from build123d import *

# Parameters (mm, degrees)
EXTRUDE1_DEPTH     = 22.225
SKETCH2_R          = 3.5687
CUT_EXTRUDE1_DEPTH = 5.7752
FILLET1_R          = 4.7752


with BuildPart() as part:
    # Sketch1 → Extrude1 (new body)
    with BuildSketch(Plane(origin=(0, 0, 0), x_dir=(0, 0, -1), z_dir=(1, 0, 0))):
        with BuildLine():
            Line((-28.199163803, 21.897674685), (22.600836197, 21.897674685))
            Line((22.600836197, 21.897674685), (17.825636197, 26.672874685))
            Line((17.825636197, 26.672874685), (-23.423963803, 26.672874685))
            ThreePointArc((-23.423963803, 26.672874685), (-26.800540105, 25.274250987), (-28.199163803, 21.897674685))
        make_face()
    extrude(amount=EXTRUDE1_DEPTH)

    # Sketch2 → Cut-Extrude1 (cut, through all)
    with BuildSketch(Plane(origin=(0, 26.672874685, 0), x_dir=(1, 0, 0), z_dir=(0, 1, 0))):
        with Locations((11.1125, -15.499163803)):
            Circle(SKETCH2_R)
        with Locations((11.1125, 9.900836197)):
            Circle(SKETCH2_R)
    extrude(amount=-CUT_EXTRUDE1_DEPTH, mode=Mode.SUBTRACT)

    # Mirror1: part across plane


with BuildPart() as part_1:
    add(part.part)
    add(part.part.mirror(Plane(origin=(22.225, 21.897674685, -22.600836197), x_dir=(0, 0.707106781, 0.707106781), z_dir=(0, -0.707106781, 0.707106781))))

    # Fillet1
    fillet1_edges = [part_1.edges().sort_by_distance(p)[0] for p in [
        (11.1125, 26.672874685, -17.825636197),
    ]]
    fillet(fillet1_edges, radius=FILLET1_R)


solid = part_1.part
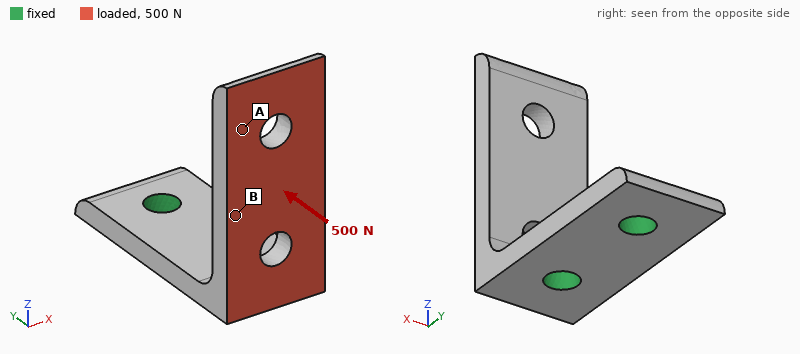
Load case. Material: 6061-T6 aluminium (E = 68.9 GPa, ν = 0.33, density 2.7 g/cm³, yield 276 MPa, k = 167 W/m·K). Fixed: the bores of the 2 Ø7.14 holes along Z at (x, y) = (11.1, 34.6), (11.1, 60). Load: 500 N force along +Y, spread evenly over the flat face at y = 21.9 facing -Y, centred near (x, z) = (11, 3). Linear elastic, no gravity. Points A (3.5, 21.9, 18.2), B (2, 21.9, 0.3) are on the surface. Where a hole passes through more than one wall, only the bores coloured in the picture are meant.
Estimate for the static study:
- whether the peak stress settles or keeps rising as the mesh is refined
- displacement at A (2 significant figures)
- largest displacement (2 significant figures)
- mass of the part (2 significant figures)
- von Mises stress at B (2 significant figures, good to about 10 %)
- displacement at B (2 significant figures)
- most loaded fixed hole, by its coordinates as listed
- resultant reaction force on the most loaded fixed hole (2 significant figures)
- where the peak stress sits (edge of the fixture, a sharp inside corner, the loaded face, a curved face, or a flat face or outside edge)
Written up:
keeps rising
0.50 mm
0.67 mm
25 g
50 MPa
0.20 mm
(11.1, 34.6)
490 N
edge of the fixture
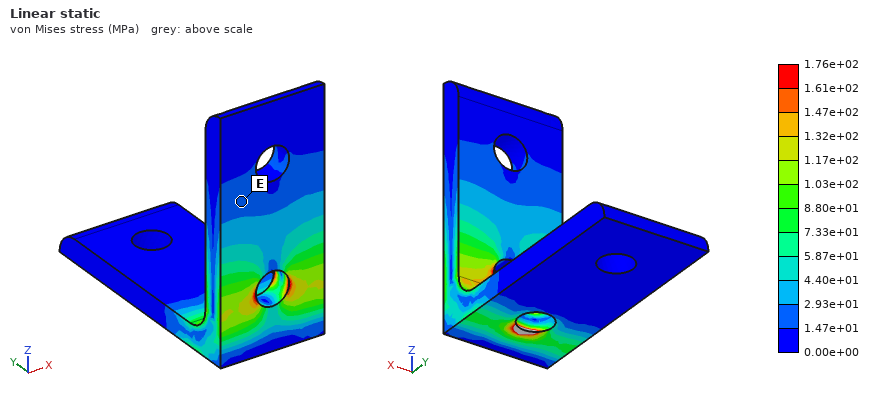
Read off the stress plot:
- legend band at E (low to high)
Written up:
1.47e+01 to 2.93e+01 MPa
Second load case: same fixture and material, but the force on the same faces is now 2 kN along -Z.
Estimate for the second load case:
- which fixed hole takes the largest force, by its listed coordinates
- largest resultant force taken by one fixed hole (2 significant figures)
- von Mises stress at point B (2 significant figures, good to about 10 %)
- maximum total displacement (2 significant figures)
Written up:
(11.1, 34.6)
2.1 kN
47 MPa
0.58 mm
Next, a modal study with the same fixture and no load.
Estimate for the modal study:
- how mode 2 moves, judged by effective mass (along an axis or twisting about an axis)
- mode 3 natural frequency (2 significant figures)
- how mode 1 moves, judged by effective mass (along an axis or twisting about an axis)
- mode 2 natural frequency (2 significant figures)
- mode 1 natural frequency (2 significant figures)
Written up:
along X
6800 Hz
along Y
3000 Hz
1500 Hz
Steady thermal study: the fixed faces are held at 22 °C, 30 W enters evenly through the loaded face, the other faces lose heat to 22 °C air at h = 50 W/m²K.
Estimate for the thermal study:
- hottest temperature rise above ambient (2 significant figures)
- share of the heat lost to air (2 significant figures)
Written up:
48 K
11 %
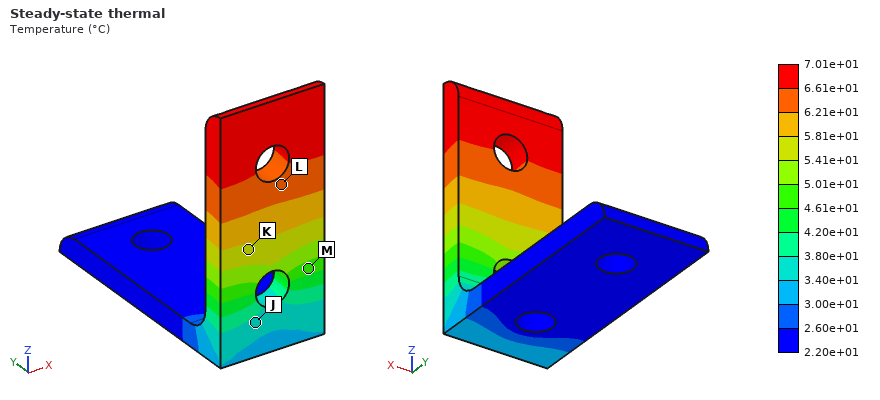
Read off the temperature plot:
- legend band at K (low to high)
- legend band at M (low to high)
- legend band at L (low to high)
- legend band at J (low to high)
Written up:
5.41e+01 to 5.81e+01 °C
4.61e+01 to 5.01e+01 °C
6.21e+01 to 6.61e+01 °C
3.40e+01 to 3.80e+01 °C
